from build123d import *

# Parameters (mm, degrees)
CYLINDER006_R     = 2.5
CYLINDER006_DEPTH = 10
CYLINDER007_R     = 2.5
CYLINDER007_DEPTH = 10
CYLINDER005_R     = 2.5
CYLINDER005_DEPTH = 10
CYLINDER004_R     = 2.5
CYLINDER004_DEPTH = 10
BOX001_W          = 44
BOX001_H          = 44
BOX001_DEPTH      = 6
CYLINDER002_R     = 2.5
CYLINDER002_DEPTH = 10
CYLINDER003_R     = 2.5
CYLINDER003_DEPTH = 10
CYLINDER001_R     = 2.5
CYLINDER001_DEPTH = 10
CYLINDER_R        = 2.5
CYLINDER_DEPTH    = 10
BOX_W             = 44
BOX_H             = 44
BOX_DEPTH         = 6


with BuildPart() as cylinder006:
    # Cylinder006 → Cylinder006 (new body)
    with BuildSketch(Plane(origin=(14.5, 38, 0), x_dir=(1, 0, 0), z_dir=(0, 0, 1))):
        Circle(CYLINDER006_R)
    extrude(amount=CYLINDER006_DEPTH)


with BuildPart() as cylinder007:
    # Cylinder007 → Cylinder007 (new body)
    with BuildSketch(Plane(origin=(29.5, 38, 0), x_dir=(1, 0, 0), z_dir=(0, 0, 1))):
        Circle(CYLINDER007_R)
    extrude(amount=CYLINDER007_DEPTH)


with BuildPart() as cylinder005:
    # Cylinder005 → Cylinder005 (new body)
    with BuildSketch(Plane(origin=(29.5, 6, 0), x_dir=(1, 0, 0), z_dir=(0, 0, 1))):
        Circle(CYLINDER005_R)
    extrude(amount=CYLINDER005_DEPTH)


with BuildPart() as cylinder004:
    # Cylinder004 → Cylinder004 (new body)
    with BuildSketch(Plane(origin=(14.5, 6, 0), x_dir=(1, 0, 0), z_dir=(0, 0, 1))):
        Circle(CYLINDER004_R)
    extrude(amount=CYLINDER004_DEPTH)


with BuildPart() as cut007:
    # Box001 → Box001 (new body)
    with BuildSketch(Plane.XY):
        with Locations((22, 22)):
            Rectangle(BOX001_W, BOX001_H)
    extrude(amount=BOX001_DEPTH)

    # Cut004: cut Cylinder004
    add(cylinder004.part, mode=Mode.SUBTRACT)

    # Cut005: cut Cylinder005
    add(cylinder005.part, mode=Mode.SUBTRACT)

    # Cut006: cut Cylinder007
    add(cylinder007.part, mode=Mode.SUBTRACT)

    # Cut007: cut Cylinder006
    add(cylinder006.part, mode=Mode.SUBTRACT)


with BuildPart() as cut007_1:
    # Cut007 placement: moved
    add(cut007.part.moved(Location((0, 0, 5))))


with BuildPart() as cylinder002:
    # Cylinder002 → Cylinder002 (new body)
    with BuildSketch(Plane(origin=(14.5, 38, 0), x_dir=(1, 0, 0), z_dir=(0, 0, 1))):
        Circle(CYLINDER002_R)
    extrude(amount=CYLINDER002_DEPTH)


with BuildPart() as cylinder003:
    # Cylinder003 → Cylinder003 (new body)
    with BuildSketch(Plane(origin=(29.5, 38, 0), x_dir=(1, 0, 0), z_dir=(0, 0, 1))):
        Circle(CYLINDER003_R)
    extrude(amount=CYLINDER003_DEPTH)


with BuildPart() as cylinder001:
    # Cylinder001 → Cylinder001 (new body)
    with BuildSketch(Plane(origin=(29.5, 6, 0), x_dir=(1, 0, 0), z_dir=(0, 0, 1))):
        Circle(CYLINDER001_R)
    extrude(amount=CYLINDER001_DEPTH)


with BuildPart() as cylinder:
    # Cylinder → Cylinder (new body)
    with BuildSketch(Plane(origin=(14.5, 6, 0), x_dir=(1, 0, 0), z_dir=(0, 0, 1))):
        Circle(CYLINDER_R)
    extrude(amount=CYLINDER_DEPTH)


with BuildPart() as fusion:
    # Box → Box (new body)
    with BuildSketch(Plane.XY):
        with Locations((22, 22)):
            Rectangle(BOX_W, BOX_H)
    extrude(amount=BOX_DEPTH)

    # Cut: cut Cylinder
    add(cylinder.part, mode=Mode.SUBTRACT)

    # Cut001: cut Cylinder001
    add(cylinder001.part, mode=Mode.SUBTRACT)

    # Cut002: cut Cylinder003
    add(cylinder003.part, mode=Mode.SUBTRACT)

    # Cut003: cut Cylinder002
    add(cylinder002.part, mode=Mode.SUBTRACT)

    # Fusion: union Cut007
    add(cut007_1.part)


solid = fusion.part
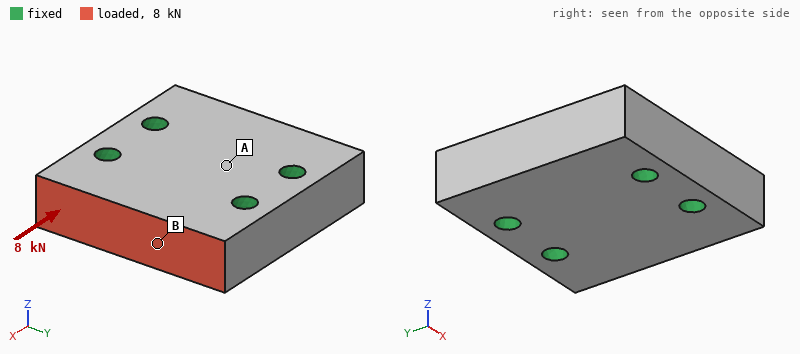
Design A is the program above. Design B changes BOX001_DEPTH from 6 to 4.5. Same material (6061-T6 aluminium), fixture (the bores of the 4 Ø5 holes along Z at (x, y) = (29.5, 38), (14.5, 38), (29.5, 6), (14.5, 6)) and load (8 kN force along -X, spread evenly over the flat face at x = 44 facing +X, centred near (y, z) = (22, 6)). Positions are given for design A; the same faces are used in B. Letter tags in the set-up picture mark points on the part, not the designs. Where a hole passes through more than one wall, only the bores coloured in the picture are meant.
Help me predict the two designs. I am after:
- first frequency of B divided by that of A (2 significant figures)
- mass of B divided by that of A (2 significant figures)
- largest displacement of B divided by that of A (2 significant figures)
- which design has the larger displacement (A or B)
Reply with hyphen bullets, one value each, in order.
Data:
- 0.93
- 0.86
- 1.2
- B
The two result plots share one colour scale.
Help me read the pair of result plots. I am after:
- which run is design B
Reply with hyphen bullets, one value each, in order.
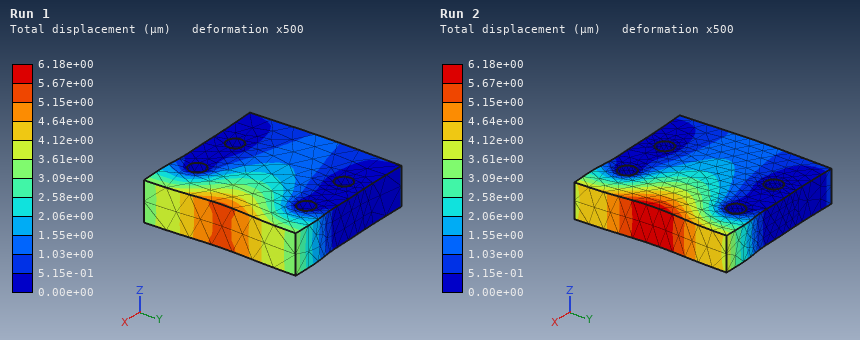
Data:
- Run 2
